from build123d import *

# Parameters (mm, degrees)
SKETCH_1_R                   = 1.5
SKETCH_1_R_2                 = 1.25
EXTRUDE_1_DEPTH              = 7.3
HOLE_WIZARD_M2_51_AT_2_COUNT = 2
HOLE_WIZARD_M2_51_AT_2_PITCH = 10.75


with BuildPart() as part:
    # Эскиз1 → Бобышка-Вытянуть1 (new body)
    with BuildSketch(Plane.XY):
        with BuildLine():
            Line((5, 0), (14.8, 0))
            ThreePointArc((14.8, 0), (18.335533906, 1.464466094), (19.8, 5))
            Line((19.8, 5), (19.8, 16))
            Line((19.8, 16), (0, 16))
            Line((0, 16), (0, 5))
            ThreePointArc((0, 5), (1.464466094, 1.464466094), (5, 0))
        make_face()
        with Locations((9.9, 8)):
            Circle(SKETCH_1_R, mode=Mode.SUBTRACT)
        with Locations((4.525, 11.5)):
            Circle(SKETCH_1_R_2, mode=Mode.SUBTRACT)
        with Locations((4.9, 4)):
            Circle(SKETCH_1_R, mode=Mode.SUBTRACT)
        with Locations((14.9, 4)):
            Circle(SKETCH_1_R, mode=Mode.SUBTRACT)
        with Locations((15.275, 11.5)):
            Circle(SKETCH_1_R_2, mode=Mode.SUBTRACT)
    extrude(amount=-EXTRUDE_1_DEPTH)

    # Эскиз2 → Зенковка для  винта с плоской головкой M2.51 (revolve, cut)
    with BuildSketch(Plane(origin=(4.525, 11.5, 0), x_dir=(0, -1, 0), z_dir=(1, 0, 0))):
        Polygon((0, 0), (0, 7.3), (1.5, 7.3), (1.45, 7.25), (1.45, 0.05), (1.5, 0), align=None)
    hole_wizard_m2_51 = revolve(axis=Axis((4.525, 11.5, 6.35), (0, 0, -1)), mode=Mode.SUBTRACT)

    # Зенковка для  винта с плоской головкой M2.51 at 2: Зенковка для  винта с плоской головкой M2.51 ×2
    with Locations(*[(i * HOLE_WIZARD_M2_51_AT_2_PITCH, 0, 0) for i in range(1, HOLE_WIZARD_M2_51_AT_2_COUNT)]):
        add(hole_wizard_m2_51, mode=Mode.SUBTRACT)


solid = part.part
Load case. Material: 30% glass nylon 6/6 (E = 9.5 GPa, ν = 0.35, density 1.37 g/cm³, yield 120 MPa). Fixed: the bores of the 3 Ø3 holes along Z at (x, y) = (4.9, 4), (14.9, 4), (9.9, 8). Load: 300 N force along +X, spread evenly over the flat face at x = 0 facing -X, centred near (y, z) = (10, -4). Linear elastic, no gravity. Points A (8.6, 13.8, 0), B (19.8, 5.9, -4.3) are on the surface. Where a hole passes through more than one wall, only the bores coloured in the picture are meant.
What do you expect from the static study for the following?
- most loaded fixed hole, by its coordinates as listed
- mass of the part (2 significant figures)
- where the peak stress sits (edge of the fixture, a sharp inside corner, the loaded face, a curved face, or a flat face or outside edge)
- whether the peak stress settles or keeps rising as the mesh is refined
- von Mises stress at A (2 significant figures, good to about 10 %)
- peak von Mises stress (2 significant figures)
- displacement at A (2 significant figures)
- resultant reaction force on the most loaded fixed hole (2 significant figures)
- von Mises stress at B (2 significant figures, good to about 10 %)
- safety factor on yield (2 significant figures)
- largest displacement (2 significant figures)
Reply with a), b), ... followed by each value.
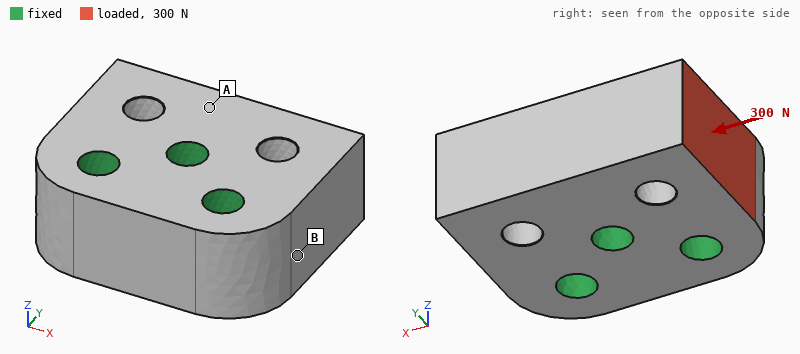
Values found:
a) (9.9, 8)
b) 2.7 g
c) a curved face
d) settles
e) 3.2 MPa
f) 14 MPa
g) 4.3 µm
h) 220 N
i) 1.2 MPa
j) 8.6
k) 9.5 µm
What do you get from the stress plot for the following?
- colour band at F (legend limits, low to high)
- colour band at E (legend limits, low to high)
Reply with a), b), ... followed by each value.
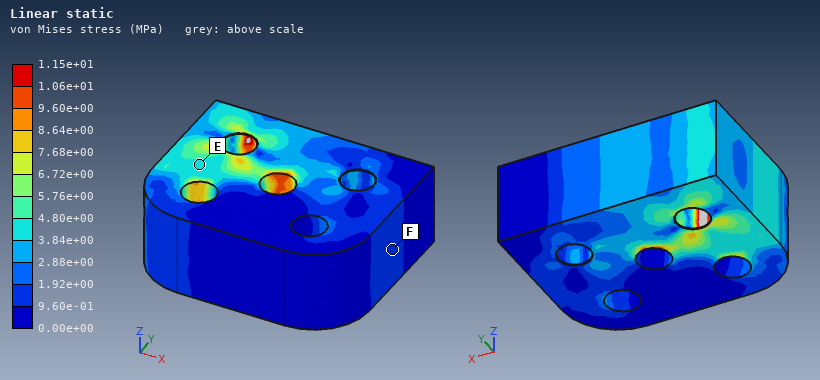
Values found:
a) 9.60e-01 to 1.92e+00 MPa
b) 3.84e+00 to 4.80e+00 MPa
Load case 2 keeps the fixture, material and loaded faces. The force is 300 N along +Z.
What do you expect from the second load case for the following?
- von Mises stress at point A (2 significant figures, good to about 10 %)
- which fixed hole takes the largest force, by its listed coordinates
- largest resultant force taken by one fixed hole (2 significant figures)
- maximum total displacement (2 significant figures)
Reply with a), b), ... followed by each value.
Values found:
a) 9.5 MPa
b) (4.9, 4)
c) 220 N
d) 39 µm
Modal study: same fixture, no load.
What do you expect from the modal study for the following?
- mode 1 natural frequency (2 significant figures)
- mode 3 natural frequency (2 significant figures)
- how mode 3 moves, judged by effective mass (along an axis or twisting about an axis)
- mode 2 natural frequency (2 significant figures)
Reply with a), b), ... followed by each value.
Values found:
a) 26 kHz
b) 30 kHz
c) along X
d) 27 kHz
